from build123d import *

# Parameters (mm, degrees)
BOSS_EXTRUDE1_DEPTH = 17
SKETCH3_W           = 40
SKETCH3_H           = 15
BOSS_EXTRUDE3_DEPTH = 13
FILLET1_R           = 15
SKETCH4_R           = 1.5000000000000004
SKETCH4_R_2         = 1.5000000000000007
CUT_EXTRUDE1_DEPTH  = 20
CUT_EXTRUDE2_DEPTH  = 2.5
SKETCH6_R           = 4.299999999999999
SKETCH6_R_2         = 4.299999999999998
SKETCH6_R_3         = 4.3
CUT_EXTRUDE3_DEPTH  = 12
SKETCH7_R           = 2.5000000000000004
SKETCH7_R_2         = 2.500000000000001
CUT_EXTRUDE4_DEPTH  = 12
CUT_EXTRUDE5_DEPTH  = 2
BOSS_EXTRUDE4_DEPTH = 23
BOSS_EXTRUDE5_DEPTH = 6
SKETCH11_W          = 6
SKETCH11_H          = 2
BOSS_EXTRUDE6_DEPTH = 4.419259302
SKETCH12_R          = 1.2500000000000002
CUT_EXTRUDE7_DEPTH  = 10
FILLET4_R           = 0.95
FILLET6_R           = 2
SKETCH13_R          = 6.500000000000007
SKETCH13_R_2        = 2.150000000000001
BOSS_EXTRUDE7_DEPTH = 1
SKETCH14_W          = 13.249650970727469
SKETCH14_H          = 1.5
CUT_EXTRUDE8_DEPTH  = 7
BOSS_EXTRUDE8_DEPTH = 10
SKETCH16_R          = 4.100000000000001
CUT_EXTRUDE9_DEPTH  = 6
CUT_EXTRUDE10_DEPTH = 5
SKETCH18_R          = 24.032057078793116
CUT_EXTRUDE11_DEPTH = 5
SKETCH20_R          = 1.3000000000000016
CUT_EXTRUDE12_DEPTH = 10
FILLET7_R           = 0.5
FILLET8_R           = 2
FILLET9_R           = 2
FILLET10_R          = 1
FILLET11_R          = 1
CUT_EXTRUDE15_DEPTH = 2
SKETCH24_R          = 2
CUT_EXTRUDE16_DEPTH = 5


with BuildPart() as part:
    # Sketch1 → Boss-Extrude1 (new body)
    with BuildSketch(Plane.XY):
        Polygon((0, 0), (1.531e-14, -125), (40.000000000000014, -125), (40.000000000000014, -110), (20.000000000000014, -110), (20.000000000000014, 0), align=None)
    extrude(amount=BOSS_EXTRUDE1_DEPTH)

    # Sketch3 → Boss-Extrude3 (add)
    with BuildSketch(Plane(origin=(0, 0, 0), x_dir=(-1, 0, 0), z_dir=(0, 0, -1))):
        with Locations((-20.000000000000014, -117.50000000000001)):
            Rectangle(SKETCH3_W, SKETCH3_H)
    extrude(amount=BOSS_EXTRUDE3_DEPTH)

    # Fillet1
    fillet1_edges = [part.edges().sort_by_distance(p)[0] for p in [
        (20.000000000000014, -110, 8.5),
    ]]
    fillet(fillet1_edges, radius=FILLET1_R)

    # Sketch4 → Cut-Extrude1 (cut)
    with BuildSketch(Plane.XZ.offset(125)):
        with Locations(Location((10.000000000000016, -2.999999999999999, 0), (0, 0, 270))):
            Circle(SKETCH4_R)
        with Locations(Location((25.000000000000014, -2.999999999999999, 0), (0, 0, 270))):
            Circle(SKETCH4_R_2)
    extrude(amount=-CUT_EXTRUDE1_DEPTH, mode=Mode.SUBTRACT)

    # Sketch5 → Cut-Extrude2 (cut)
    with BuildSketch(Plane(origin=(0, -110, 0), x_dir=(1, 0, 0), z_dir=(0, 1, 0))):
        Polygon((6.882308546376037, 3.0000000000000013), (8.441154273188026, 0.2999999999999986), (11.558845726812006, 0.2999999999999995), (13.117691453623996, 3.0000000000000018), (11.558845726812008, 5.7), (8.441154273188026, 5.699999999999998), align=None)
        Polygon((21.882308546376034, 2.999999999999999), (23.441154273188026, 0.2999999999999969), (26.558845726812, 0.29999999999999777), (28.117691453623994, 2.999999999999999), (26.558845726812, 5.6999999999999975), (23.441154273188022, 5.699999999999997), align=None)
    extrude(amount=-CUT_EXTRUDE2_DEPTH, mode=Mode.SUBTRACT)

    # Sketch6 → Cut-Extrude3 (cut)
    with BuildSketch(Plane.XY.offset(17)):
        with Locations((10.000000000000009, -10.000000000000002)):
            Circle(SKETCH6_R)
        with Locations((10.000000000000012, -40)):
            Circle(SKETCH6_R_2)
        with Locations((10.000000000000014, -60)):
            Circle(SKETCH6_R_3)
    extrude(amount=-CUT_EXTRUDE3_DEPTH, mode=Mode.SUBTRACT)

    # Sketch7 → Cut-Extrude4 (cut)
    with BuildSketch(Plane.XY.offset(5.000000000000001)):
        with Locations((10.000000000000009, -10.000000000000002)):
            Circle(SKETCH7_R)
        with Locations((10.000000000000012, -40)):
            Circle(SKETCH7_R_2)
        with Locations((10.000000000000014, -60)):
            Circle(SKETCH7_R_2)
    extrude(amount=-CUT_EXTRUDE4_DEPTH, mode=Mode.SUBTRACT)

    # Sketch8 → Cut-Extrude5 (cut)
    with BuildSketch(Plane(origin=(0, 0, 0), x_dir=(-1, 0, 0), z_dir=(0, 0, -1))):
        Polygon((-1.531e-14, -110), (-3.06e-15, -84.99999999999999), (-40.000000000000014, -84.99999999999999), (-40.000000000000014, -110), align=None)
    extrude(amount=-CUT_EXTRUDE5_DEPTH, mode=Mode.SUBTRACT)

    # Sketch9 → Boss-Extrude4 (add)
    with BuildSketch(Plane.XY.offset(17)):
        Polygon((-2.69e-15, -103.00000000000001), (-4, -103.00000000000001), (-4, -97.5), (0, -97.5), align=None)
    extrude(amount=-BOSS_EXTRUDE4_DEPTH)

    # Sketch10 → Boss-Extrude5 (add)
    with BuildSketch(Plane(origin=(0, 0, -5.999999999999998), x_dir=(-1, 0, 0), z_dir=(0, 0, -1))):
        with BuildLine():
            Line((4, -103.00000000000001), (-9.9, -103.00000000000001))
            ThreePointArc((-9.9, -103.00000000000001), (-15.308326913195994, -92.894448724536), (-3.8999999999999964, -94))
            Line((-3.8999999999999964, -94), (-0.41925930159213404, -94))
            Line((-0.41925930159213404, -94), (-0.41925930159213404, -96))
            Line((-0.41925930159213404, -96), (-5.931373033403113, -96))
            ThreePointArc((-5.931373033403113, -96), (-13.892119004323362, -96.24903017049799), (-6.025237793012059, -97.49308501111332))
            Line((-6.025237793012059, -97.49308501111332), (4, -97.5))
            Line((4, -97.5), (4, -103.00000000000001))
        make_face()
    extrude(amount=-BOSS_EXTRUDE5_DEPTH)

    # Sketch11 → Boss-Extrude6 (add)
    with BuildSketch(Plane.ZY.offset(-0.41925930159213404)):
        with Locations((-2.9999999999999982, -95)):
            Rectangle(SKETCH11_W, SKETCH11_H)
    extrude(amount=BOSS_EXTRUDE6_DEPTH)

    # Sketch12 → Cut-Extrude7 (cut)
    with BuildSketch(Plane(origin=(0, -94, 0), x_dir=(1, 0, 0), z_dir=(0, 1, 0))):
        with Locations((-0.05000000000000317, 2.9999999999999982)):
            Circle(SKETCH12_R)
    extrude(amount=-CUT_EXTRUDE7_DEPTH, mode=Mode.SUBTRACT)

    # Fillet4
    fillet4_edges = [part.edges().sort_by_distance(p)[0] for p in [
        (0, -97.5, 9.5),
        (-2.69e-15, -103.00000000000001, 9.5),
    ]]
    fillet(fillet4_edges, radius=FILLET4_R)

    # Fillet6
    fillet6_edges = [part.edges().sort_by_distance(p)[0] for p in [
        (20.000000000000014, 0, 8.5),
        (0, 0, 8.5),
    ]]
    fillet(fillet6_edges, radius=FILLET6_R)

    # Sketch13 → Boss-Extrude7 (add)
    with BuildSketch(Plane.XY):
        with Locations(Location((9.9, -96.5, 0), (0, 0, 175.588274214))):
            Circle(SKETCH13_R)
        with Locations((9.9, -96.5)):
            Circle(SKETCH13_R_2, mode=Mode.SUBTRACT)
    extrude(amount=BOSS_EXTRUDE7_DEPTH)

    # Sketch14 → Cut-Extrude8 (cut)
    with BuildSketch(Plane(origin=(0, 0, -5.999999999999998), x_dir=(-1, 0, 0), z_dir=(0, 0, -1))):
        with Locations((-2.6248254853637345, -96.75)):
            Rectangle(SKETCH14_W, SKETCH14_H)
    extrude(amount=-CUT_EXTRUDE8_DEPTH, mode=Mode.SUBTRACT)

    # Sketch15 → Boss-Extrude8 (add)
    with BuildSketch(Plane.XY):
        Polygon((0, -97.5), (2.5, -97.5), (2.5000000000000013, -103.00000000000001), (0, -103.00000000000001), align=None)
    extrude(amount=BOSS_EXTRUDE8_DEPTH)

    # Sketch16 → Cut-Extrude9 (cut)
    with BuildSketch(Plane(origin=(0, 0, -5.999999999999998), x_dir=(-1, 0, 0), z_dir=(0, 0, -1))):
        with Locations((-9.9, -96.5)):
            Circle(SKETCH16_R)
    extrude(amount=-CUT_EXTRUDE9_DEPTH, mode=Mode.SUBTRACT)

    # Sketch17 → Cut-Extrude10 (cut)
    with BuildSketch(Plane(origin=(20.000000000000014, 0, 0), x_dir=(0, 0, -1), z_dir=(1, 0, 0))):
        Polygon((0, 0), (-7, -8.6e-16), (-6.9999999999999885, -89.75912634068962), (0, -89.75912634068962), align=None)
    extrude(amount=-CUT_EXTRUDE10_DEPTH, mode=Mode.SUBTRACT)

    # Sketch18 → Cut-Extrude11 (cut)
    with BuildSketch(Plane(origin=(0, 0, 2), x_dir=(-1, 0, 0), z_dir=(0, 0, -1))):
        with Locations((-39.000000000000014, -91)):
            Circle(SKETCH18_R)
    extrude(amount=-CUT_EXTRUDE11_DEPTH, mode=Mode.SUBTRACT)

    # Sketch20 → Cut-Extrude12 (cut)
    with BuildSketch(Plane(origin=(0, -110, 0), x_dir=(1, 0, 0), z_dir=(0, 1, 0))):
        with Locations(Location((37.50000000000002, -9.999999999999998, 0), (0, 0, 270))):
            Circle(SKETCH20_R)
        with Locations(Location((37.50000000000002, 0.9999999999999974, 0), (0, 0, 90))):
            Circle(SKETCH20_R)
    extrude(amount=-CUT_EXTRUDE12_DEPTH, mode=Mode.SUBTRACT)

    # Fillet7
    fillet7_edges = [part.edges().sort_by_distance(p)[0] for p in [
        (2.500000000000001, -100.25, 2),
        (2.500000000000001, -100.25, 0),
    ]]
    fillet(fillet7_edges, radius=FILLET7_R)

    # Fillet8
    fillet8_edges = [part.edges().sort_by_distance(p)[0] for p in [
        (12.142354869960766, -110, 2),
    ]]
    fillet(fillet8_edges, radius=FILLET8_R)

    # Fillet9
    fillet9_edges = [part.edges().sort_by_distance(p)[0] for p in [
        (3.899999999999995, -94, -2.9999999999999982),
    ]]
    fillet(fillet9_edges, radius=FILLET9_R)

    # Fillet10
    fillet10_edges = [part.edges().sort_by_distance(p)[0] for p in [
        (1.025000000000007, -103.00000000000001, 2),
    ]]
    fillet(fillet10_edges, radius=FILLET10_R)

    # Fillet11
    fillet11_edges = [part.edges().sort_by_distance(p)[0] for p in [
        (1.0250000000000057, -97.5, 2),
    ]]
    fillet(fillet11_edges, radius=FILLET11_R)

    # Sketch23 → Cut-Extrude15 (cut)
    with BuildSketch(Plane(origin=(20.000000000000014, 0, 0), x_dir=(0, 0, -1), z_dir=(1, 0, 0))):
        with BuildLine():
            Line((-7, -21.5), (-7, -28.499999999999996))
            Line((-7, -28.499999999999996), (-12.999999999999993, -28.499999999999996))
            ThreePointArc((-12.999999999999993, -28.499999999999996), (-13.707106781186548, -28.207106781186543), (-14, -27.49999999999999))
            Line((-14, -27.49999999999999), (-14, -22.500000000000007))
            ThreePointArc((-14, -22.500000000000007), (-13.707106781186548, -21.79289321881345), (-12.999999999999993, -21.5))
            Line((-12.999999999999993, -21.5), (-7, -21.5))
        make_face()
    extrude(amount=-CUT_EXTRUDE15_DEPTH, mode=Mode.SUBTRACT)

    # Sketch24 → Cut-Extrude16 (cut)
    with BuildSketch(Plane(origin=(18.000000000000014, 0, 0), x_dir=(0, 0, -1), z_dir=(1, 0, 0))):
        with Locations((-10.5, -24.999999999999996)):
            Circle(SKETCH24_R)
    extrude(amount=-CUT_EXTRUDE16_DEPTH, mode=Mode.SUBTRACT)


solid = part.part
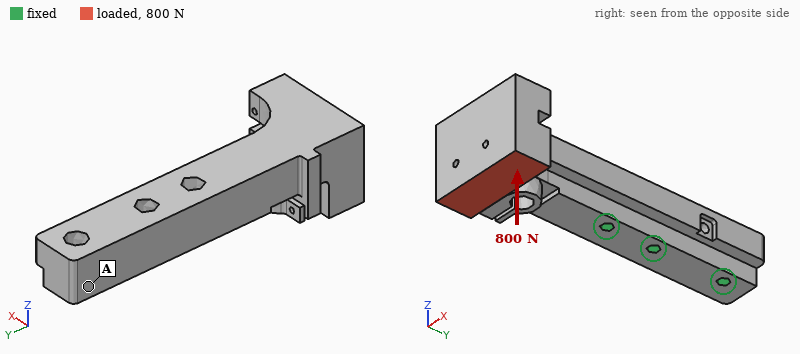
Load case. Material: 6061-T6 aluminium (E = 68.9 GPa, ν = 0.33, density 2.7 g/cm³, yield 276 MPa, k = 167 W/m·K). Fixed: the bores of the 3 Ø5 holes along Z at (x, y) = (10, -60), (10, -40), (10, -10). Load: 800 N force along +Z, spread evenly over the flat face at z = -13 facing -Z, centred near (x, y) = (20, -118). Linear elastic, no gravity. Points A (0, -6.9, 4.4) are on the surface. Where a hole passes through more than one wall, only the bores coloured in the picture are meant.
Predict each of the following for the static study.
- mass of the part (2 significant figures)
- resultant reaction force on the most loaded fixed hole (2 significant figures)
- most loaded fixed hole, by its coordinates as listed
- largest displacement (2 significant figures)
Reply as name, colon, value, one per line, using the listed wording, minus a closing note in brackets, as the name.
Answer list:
mass of the part: 130 g
resultant reaction force on the most loaded fixed hole: 2.9 kN
most loaded fixed hole, by its coordinates as listed: (10, -60)
largest displacement: 0.29 mm
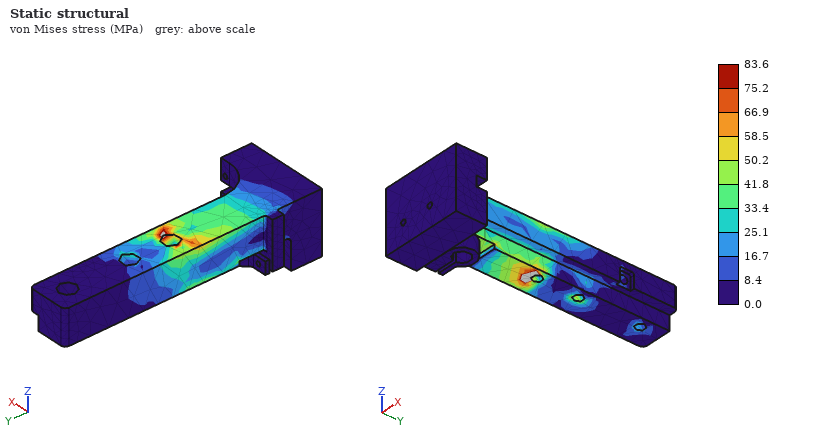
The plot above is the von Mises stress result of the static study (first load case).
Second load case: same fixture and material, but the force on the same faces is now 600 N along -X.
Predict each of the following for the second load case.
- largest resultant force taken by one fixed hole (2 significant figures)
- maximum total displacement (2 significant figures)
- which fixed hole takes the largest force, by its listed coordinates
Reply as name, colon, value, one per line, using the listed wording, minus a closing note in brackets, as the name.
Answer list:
largest resultant force taken by one fixed hole: 1.7 kN
maximum total displacement: 0.22 mm
which fixed hole takes the largest force, by its listed coordinates: (10, -60)
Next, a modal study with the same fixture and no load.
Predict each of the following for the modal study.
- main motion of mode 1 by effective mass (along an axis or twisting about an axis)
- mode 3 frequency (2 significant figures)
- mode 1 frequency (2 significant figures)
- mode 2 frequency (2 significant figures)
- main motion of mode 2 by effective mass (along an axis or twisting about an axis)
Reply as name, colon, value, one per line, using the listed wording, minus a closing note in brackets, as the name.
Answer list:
main motion of mode 1 by effective mass: along Z
mode 3 frequency: 2900 Hz
mode 1 frequency: 1300 Hz
mode 2 frequency: 1500 Hz
main motion of mode 2 by effective mass: along X
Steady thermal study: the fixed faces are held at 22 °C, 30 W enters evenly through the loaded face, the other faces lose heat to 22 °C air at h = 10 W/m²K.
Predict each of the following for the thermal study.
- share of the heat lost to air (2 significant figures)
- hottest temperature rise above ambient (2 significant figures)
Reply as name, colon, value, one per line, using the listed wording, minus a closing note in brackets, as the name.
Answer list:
share of the heat lost to air: 8.8 %
hottest temperature rise above ambient: 43 K
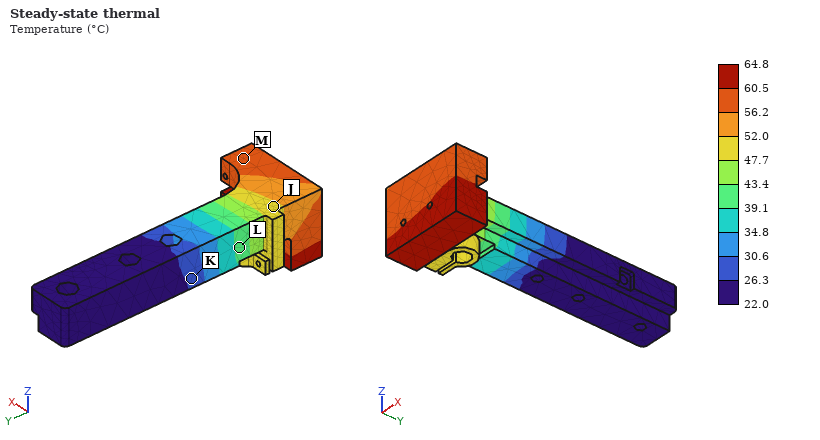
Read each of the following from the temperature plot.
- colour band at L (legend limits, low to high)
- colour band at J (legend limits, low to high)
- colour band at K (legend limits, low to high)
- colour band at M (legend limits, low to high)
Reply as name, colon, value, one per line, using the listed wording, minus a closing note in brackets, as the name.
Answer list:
colour band at L: 39.1 to 43.4 °C
colour band at J: 47.7 to 52.0 °C
colour band at K: 26.3 to 30.6 °C
colour band at M: 56.2 to 60.5 °C
